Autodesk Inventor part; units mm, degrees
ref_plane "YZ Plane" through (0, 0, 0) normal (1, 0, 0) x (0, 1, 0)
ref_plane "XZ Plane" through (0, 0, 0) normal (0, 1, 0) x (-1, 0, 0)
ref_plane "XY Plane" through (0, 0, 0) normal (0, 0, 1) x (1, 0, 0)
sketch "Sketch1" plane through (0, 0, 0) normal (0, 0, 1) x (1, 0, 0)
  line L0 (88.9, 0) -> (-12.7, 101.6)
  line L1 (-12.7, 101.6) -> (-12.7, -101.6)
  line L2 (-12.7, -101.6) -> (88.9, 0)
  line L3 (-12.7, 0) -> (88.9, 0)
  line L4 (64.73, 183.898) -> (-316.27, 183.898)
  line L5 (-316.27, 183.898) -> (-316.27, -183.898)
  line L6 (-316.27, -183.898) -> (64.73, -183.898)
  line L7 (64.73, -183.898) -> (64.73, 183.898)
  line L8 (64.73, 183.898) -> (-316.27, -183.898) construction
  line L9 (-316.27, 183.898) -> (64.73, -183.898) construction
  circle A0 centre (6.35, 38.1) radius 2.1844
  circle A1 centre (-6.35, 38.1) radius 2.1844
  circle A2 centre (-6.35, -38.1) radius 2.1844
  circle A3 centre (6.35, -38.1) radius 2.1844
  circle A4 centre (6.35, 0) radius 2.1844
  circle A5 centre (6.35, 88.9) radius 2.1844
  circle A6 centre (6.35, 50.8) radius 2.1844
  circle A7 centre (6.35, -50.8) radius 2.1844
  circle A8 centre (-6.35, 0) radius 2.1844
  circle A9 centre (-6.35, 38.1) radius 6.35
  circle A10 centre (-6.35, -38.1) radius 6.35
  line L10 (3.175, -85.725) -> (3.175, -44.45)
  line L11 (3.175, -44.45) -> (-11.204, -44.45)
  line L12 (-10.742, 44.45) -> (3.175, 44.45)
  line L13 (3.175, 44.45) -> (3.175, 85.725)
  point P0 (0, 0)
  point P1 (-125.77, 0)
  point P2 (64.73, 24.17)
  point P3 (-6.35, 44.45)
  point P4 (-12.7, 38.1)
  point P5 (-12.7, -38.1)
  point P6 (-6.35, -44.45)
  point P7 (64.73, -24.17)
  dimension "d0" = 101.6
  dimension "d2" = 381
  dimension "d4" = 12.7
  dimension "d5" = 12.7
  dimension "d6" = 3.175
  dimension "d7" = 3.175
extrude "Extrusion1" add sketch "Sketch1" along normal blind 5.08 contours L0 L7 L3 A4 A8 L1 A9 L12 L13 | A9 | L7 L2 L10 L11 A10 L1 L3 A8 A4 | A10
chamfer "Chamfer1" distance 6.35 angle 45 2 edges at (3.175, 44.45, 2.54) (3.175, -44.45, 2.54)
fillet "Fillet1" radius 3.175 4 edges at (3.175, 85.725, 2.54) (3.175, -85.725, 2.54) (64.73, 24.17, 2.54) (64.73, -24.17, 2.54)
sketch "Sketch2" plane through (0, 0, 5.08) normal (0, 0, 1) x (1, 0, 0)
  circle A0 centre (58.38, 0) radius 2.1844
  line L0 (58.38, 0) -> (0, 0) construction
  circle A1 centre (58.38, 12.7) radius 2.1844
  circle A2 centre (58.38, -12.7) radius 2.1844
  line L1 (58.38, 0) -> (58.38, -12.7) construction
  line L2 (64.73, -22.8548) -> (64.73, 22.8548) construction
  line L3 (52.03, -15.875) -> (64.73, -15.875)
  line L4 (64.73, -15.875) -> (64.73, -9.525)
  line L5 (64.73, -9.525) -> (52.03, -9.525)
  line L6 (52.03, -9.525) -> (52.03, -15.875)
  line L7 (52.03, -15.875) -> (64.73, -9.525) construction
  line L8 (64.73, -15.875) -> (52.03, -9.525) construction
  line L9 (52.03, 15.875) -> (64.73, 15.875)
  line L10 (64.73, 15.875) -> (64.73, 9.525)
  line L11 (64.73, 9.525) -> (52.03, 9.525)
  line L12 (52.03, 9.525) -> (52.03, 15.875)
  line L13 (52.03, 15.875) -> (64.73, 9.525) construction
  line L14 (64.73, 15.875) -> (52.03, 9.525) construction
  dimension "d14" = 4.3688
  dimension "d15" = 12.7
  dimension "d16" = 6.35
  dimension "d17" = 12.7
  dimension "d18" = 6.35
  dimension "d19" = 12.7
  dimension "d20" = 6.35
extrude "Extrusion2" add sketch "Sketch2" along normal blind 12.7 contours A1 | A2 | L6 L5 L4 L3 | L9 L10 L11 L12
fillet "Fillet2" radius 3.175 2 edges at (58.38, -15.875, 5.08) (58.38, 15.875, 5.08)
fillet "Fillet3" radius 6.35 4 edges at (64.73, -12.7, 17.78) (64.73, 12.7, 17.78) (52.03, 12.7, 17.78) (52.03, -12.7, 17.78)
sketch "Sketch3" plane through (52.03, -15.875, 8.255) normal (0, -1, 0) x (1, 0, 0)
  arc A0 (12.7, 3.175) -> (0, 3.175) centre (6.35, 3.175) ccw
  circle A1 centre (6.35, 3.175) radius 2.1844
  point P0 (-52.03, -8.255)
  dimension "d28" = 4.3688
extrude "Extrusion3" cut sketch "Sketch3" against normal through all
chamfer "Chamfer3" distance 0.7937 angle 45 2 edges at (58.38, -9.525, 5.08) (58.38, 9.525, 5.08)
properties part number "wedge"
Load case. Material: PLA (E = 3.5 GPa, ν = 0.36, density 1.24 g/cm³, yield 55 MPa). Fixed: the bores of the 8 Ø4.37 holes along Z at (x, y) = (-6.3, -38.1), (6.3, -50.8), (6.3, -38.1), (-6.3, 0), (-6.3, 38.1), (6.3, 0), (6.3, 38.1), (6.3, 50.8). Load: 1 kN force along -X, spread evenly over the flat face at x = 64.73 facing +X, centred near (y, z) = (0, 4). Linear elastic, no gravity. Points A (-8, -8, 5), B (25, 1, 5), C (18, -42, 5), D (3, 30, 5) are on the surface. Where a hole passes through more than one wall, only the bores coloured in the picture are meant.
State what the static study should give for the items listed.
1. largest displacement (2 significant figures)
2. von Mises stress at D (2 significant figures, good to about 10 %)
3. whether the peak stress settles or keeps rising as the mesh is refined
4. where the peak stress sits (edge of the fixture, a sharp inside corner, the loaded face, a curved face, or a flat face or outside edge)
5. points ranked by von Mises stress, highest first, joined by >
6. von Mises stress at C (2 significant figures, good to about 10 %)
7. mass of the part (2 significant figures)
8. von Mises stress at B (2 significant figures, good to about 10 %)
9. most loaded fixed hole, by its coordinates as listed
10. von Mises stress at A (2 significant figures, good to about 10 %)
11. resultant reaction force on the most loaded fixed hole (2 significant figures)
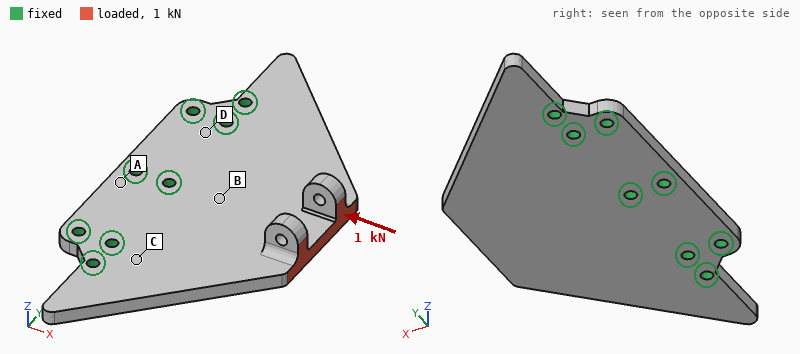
0.72 mm
2.5 MPa
keeps rising
edge of the fixture
B > C > D > A
4.1 MPa
53 g
6.3 MPa
(6.3, 0)
1.0 MPa
310 N
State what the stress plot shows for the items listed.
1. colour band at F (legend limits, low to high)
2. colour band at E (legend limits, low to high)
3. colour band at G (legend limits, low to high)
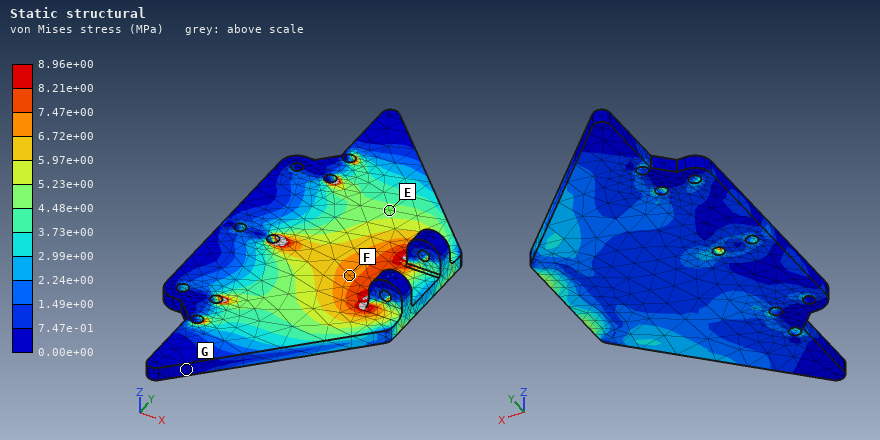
6.72e+00 to 7.47e+00 MPa
4.48e+00 to 5.23e+00 MPa
0.00e+00 to 7.47e-01 MPa
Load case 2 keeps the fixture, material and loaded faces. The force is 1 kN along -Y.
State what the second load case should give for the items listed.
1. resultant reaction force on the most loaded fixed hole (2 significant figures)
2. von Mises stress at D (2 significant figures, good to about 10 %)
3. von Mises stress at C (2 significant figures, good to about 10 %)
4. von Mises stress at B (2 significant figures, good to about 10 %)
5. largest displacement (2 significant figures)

380 N
1.3 MPa
4.0 MPa
4.2 MPa
0.31 mm
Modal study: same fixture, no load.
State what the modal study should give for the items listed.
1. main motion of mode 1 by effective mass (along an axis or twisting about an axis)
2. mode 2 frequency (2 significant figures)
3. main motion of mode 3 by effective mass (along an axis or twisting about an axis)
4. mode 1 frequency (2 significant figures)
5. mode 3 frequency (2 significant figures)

along Z
1000 Hz
along Z
450 Hz
1800 Hz
